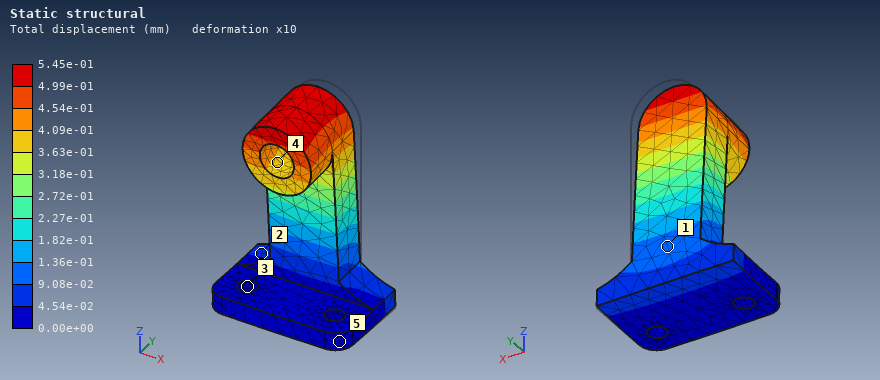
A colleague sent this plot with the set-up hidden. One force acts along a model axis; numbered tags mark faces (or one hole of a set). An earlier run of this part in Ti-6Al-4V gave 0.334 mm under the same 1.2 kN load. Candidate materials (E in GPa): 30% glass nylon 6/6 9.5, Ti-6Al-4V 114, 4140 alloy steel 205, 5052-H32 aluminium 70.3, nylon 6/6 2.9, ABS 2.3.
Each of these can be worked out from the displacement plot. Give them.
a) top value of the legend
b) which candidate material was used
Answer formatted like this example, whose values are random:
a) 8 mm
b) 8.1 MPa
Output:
a) 5.45e-01 mm
b) 5052-H32 aluminium
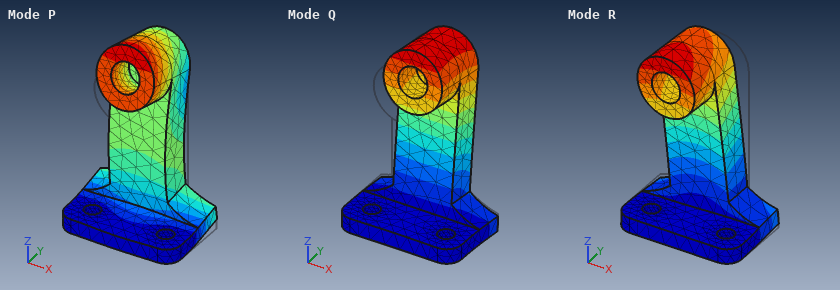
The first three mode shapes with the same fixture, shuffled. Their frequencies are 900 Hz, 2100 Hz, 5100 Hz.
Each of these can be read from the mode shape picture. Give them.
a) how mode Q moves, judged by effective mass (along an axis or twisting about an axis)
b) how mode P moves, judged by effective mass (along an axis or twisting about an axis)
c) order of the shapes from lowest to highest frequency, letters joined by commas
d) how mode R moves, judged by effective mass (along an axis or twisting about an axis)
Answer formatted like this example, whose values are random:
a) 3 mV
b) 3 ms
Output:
a) along Y
b) along Z
c) Q, R, P
d) along X
